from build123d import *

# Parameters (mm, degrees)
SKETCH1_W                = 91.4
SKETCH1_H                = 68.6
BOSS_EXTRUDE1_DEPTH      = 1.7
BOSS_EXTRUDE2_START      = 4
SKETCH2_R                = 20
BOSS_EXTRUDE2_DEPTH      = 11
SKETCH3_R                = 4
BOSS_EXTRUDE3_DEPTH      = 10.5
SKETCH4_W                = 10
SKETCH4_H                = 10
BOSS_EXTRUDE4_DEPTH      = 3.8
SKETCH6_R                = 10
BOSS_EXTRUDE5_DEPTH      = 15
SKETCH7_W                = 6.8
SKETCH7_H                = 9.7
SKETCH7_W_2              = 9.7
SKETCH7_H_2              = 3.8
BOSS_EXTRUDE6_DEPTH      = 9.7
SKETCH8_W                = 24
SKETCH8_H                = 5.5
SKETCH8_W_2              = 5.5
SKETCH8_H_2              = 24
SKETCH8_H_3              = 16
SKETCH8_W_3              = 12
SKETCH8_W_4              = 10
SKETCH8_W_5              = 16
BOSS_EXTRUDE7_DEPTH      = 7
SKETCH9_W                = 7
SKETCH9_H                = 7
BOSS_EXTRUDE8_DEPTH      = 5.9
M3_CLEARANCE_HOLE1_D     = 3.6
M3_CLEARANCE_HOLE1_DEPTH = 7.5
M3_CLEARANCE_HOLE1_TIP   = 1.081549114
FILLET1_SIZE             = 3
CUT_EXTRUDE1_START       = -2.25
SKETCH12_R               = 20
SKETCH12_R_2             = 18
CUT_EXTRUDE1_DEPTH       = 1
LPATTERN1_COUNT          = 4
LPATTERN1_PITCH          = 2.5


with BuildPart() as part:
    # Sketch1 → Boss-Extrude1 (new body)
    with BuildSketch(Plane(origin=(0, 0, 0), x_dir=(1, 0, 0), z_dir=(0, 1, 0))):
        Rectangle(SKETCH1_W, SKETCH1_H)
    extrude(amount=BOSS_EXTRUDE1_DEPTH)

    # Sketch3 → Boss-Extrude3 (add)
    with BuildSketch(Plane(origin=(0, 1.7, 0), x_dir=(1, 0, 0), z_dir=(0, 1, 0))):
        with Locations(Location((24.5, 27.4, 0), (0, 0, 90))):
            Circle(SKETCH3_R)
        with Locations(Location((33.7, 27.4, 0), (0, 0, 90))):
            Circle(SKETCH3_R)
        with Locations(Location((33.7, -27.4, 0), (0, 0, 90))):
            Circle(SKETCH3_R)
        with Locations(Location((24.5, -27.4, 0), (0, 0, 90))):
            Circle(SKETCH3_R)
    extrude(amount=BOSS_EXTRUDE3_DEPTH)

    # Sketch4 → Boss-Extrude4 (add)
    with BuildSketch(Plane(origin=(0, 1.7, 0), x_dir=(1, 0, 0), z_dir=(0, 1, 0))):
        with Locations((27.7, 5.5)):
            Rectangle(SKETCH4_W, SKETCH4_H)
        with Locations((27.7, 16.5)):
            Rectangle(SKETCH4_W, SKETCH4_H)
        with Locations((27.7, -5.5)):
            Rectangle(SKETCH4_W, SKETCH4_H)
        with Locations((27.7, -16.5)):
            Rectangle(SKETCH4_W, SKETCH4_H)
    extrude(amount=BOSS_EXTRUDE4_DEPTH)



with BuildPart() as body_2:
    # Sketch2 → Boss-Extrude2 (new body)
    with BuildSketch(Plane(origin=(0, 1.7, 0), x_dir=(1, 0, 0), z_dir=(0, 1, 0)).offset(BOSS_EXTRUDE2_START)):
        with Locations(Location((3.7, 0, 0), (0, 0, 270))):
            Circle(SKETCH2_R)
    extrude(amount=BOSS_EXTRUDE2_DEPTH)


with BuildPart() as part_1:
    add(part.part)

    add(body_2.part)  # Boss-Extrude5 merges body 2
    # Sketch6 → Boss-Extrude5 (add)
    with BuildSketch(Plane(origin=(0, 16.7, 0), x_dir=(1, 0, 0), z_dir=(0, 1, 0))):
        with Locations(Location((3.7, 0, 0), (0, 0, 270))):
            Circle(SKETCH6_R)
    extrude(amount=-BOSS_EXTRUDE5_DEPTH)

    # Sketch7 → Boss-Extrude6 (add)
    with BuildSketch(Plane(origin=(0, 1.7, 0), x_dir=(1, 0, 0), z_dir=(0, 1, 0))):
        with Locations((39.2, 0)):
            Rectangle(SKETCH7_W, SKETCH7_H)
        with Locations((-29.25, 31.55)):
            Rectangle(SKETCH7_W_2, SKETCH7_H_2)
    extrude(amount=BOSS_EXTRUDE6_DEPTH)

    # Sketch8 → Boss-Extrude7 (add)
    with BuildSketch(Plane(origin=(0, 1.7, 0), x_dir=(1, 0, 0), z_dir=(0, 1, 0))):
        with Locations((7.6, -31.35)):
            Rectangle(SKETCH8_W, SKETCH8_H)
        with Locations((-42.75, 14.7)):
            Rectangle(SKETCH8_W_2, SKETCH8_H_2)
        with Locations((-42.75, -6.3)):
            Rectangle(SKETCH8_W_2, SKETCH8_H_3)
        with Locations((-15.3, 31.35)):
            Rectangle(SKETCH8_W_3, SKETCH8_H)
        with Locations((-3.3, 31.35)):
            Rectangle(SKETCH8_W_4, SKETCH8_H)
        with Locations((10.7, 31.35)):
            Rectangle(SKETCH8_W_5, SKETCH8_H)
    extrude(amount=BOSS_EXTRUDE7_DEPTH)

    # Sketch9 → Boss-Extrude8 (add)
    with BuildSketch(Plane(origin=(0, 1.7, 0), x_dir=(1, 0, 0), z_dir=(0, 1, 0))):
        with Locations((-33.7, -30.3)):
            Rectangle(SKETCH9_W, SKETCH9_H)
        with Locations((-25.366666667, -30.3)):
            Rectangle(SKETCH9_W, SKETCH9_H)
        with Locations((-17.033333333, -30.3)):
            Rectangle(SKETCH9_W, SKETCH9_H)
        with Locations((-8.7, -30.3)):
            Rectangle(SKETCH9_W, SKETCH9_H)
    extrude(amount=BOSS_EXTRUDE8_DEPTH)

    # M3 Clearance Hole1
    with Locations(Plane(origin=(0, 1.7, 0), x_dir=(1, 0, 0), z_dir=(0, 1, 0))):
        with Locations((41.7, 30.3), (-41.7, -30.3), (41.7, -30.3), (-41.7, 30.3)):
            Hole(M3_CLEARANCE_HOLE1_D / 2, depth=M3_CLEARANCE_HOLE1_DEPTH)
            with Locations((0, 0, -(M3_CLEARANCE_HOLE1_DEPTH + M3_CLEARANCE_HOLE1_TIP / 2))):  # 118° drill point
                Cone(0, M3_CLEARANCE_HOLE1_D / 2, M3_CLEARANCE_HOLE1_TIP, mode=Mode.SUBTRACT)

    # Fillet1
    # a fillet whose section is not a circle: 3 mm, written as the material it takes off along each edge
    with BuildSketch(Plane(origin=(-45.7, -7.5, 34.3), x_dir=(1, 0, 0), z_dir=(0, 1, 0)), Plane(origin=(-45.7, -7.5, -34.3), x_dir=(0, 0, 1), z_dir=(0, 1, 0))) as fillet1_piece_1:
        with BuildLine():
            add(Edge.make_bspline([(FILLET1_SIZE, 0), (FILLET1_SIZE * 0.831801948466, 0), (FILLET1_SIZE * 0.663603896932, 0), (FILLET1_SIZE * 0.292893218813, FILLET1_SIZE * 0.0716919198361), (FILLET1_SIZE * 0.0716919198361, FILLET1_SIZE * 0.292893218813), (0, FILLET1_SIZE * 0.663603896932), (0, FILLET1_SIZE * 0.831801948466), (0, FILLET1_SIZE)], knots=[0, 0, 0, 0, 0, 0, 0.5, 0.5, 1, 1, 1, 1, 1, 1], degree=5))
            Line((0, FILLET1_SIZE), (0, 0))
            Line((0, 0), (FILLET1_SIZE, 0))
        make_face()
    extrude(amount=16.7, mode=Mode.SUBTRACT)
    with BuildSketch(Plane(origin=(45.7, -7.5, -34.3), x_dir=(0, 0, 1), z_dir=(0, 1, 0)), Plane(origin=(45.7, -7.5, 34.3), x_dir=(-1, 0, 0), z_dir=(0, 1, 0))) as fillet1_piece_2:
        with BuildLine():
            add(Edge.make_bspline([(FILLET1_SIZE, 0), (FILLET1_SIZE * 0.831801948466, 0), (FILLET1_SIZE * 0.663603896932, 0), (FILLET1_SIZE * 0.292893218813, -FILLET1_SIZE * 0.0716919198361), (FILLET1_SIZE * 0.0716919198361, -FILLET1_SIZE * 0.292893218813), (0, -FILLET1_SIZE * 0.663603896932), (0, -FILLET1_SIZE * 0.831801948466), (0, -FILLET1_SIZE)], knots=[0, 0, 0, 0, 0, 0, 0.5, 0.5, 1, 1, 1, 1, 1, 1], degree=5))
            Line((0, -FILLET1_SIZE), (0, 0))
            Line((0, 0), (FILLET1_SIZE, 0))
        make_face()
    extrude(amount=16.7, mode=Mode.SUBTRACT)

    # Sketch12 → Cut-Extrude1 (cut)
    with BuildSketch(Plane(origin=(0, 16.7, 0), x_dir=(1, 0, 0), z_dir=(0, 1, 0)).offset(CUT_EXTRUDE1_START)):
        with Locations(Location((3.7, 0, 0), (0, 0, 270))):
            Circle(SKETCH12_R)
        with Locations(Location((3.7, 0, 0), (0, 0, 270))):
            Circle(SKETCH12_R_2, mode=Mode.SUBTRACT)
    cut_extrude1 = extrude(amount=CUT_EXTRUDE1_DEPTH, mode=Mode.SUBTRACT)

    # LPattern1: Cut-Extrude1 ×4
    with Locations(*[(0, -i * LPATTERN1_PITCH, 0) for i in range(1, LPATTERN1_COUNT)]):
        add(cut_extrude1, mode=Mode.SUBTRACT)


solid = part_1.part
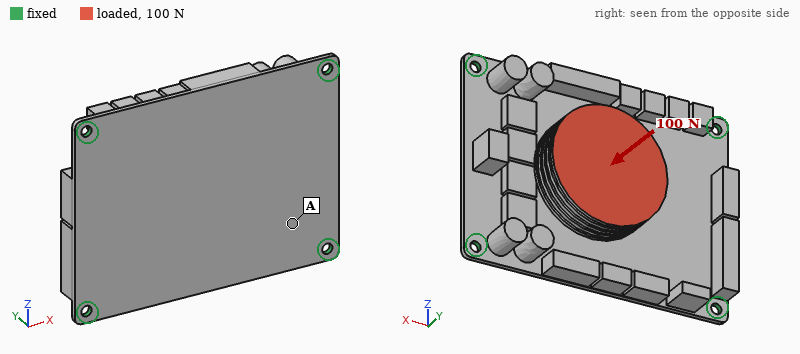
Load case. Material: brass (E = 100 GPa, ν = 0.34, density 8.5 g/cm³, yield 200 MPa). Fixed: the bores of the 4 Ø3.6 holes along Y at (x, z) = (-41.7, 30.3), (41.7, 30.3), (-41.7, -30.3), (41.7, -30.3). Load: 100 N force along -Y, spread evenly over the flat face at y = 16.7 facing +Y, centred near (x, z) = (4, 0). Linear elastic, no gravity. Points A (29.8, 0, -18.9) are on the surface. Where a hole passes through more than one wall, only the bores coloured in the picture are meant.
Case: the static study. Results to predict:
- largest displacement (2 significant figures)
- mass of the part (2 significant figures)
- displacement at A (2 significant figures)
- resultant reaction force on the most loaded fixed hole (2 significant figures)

89 µm
290 g
30 µm
33 N
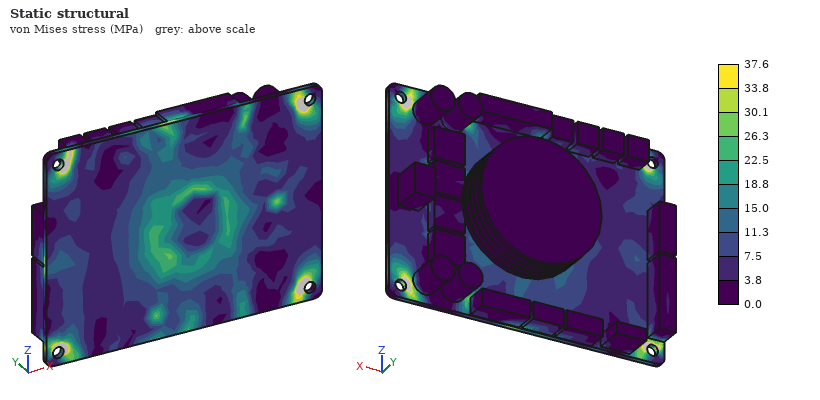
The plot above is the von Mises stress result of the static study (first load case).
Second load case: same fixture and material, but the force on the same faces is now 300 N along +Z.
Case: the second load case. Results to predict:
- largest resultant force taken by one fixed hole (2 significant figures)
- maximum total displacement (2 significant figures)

160 N
0.15 mm
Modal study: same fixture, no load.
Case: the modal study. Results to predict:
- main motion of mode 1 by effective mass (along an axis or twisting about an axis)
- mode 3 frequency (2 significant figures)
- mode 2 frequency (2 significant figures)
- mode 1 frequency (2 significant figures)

along Y
870 Hz
780 Hz
430 Hz
